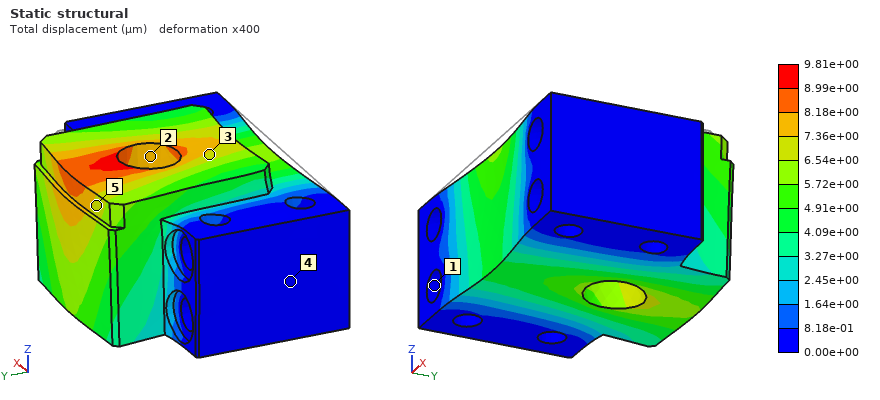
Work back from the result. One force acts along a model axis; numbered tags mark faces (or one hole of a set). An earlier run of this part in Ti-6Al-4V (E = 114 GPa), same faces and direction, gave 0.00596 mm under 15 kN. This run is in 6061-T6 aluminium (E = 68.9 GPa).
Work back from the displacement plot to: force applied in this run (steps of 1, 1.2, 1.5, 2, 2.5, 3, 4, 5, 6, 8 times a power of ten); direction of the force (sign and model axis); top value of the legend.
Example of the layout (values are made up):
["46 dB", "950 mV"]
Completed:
["15 kN", "+Y", "9.81e+00 µm"]
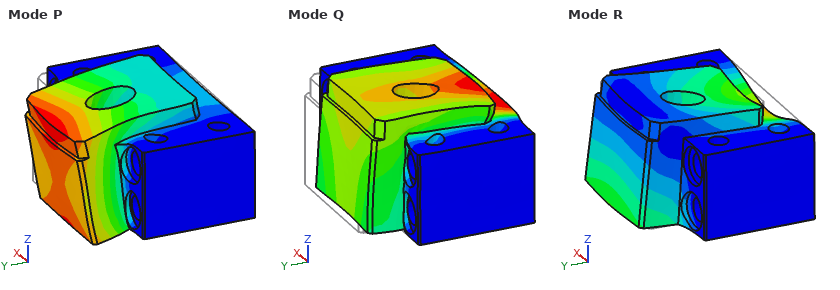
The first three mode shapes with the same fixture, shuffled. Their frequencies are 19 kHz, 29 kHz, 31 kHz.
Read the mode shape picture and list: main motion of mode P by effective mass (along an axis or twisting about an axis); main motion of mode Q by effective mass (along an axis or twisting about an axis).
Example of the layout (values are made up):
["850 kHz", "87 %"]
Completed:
["along Z", "along Y"]
